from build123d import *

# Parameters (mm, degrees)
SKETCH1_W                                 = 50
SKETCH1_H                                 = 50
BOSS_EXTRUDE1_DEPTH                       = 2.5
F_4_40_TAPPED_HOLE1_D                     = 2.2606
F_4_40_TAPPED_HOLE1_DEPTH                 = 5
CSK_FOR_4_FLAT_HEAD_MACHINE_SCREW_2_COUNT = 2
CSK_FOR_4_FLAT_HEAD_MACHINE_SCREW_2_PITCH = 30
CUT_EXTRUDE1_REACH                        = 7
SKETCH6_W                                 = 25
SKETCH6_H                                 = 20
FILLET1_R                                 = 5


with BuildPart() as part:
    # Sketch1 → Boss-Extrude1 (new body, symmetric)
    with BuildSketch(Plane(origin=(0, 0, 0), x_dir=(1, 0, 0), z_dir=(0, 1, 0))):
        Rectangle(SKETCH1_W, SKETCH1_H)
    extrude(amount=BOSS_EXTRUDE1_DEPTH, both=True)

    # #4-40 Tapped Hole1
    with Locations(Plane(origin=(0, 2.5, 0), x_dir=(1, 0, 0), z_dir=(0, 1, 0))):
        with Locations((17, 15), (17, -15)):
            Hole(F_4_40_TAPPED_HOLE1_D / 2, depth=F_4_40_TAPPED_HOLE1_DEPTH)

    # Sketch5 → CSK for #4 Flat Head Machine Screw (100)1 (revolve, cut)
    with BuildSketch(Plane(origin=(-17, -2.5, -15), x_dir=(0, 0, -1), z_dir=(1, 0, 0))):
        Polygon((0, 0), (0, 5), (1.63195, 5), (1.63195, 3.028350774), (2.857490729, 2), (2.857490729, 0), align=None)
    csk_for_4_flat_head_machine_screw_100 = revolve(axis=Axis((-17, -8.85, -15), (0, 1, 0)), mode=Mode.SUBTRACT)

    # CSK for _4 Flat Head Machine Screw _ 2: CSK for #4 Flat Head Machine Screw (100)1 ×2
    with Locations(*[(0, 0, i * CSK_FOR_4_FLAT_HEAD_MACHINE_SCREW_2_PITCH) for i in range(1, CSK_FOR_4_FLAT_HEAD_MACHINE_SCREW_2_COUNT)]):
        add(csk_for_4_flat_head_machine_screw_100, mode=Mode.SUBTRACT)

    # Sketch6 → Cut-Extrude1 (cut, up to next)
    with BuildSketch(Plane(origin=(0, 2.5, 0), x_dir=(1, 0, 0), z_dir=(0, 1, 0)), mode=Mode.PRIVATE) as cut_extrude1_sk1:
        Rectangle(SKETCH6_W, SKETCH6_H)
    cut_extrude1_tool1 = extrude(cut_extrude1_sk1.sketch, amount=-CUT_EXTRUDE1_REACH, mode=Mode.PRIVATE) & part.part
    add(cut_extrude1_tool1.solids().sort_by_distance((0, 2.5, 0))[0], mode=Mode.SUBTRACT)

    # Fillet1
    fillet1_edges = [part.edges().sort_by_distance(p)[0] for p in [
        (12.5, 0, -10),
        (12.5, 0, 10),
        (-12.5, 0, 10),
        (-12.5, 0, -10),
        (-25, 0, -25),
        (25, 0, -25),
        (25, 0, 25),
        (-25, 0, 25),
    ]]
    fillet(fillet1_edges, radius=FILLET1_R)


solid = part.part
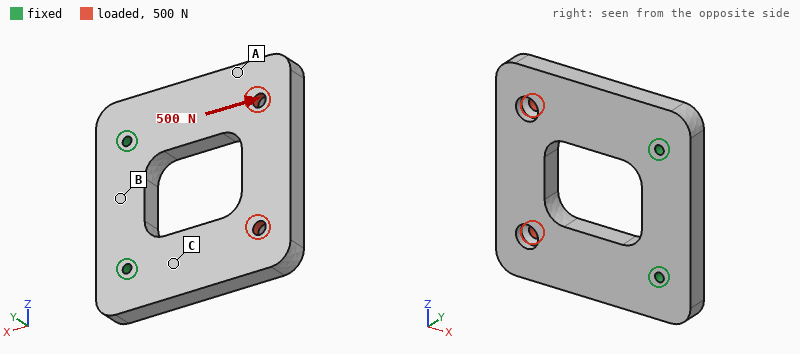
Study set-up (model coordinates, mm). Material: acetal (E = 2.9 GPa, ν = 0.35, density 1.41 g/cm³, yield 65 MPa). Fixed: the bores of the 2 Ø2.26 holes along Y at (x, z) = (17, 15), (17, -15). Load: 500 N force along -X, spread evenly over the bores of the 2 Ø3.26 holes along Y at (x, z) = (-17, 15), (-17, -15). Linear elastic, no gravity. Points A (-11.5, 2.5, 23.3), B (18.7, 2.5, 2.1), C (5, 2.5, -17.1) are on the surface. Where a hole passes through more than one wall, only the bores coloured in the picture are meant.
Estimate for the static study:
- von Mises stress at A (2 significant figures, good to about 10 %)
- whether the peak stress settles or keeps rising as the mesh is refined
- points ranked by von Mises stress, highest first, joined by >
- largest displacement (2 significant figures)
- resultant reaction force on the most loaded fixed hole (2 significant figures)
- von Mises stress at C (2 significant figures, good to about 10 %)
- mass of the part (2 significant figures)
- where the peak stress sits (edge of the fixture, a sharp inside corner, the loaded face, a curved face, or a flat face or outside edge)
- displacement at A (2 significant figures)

6.0 MPa
keeps rising
C > A > B
0.75 mm
250 N
9.4 MPa
14 g
edge of the fixture
0.37 mm
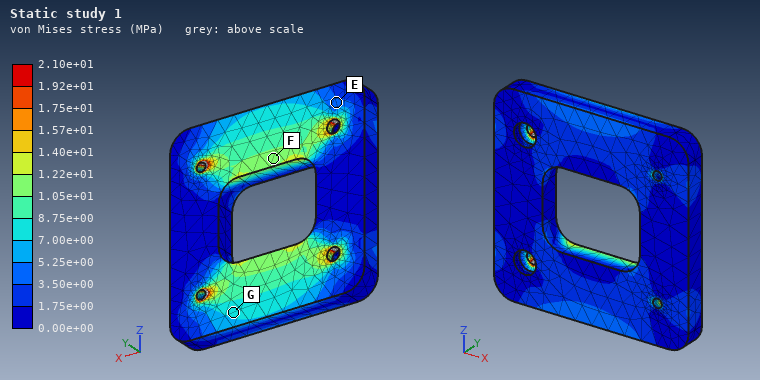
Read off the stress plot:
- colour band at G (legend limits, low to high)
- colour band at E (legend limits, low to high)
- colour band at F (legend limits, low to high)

7.00e+00 to 8.75e+00 MPa
3.50e+00 to 5.25e+00 MPa
1.05e+01 to 1.22e+01 MPa
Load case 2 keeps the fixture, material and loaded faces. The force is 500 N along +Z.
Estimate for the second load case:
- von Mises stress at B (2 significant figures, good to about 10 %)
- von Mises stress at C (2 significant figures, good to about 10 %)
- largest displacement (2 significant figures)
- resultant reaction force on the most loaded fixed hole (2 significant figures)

12 MPa
12 MPa
0.74 mm
570 N
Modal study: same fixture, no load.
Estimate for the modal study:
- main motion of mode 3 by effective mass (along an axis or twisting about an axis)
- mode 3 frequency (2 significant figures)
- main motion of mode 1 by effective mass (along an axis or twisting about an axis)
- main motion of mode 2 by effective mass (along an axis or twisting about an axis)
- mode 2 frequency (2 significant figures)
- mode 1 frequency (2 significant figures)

along Z
1900 Hz
along Y
twisting about X
1100 Hz
520 Hz
